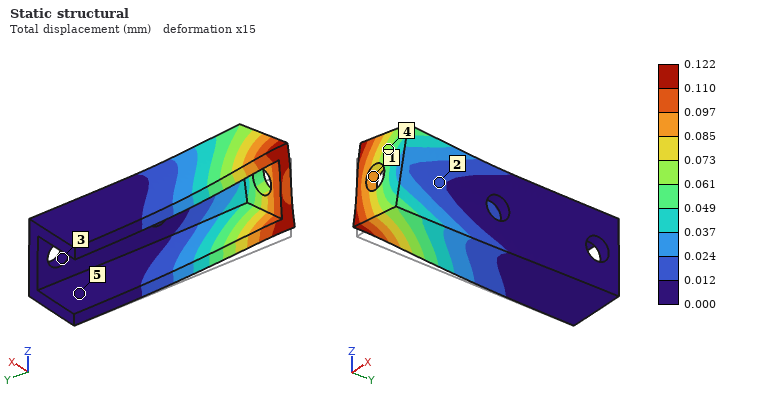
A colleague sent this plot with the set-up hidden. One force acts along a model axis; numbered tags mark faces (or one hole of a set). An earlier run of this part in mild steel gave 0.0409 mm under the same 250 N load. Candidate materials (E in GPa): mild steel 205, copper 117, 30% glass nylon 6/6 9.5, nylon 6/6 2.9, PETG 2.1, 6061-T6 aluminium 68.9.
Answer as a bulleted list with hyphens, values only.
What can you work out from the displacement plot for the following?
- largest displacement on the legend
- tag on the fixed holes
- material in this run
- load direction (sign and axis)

- 0.122 mm
- 3
- 6061-T6 aluminium
- +Z
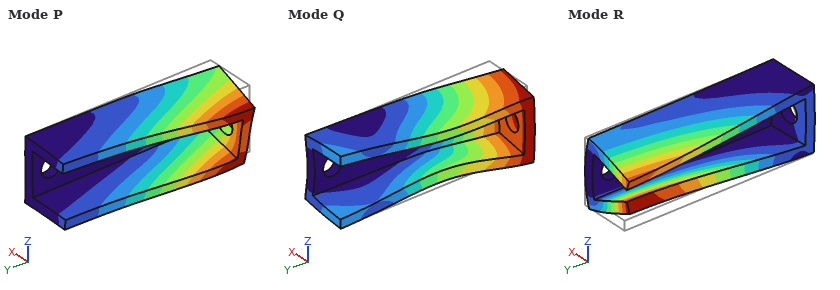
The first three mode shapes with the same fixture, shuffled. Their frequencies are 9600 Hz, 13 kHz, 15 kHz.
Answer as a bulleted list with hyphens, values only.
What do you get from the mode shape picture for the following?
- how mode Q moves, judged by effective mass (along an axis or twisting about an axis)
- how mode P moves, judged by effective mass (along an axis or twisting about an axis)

- along X
- along Z
